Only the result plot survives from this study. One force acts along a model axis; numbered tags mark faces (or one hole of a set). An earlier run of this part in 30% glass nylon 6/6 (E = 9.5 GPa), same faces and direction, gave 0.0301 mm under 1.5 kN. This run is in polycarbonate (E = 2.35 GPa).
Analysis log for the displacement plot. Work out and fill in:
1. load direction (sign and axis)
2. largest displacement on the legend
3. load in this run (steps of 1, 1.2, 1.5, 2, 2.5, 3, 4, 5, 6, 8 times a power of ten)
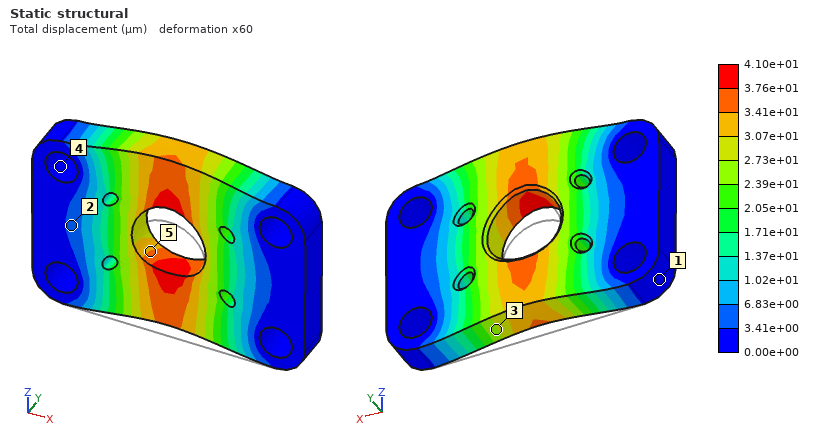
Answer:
+Z
4.10e+01 µm
500 N
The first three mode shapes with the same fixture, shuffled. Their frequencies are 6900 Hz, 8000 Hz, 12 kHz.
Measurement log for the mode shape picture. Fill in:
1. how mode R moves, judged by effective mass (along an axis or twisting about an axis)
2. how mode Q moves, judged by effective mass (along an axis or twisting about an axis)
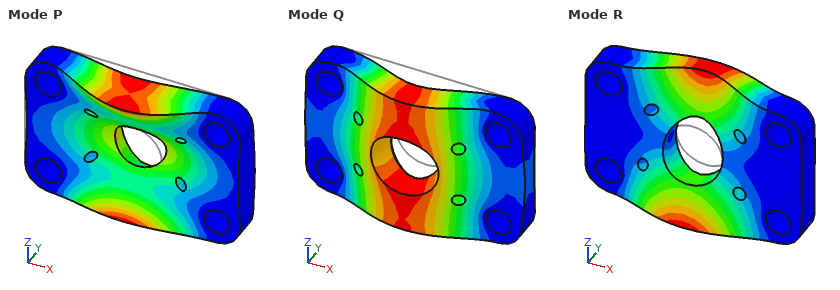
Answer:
twisting about X
along Y
